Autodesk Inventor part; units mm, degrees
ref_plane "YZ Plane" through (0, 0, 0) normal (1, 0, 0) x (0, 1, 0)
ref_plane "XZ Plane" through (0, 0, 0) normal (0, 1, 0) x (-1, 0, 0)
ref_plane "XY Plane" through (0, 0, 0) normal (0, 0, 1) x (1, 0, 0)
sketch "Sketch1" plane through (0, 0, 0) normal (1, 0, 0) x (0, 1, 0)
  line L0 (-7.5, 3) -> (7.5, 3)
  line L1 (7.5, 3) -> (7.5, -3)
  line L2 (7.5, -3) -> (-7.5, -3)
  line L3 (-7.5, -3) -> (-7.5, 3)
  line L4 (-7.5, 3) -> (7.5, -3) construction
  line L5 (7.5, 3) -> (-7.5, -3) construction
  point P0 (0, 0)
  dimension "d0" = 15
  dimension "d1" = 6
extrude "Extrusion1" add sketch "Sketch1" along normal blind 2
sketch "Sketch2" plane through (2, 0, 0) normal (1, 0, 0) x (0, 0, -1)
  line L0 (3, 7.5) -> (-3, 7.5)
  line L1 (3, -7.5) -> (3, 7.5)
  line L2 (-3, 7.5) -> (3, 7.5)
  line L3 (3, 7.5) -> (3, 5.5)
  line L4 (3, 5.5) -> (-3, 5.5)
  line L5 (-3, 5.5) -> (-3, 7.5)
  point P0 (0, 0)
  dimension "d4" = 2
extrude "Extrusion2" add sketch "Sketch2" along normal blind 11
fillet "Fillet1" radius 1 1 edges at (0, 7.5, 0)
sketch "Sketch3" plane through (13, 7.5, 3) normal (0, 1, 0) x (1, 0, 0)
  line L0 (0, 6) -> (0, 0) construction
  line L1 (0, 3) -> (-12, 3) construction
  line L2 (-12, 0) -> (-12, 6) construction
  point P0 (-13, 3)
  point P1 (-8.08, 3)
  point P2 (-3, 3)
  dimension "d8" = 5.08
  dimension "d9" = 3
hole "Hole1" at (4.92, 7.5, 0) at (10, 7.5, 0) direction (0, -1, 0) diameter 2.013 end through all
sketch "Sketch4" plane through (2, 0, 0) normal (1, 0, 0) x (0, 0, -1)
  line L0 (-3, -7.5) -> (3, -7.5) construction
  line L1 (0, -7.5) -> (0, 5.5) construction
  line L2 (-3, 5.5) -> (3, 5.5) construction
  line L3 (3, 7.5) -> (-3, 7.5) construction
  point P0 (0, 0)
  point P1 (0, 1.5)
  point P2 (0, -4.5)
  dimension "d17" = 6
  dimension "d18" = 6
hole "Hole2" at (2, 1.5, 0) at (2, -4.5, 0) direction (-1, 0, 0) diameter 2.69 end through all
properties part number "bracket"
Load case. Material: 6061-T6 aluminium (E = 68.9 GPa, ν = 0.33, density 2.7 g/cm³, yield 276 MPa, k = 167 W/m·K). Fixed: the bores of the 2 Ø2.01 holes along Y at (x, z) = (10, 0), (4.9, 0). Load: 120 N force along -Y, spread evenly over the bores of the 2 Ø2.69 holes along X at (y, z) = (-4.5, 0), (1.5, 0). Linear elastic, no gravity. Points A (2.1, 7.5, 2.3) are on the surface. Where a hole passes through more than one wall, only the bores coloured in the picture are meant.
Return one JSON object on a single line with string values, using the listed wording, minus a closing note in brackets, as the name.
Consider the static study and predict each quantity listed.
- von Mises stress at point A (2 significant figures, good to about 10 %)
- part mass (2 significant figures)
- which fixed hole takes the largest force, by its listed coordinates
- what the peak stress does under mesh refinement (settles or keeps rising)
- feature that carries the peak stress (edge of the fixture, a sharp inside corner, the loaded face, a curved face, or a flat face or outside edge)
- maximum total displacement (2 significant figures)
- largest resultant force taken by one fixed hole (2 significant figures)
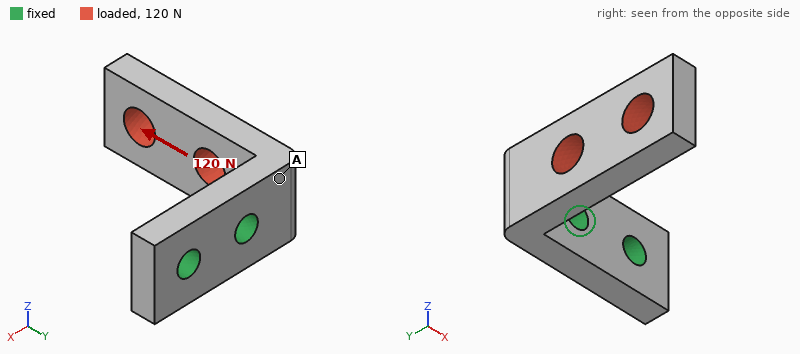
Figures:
{"von Mises stress at point A": "26 MPa", "part mass": "0.74 g", "which fixed hole takes the largest force, by its listed coordinates": "(4.9, 0)", "what the peak stress does under mesh refinement": "keeps rising", "feature that carries the peak stress": "edge of the fixture", "maximum total displacement": "41 µm", "largest resultant force taken by one fixed hole": "130 N"}
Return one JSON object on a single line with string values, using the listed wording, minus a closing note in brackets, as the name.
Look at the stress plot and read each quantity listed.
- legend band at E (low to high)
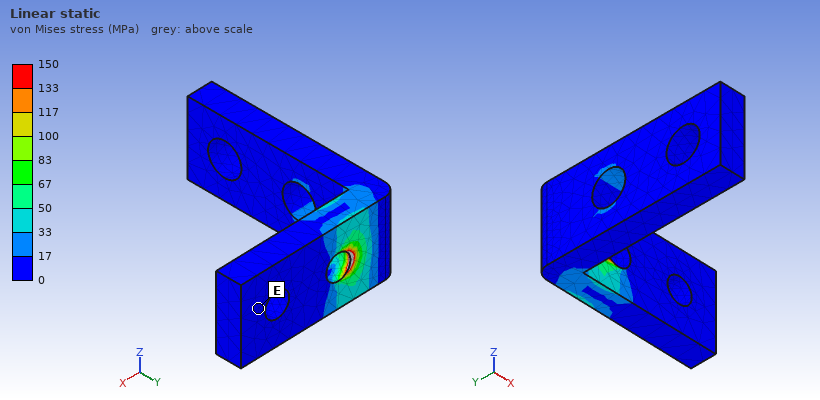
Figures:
{"legend band at E": "0 to 17 MPa"}
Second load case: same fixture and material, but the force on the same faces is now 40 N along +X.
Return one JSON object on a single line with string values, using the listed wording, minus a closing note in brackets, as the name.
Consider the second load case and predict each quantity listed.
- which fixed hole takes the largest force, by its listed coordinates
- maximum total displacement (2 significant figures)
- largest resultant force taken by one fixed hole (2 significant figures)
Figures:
{"which fixed hole takes the largest force, by its listed coordinates": "(4.9, 0)", "maximum total displacement": "0.11 mm", "largest resultant force taken by one fixed hole": "38 N"}
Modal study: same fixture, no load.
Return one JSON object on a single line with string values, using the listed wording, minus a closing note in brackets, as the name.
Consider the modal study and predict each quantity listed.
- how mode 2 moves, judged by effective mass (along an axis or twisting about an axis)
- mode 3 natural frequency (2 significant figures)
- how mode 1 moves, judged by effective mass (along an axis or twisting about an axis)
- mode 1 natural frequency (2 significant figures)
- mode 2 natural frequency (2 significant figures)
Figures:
{"how mode 2 moves, judged by effective mass": "along Z", "mode 3 natural frequency": "28 kHz", "how mode 1 moves, judged by effective mass": "along X", "mode 1 natural frequency": "6300 Hz", "mode 2 natural frequency": "10 kHz"}
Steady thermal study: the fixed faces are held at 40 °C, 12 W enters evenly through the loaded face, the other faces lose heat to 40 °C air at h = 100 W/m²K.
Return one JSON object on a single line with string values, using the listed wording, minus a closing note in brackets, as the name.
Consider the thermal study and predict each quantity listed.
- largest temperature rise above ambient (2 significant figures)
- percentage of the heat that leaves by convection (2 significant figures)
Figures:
{"largest temperature rise above ambient": "72 K", "percentage of the heat that leaves by convection": "9.5 %"}
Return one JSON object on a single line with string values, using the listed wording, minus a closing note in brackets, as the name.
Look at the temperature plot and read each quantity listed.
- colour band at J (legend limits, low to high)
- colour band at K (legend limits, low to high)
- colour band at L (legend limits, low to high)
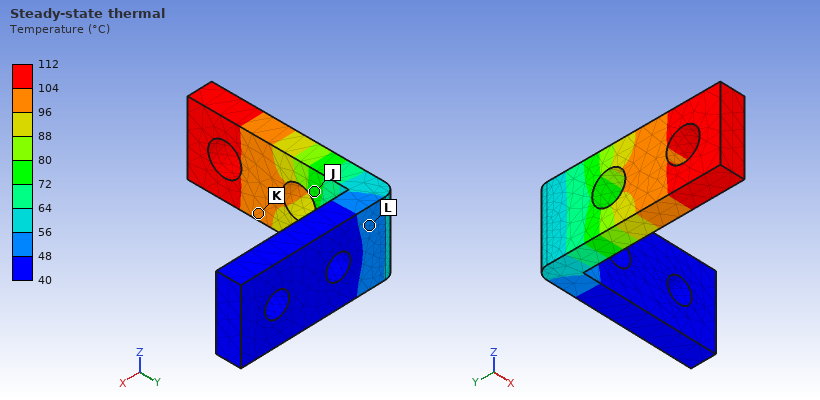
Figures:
{"colour band at J": "72 to 80 °C", "colour band at K": "96 to 104 °C", "colour band at L": "48 to 56 °C"}
